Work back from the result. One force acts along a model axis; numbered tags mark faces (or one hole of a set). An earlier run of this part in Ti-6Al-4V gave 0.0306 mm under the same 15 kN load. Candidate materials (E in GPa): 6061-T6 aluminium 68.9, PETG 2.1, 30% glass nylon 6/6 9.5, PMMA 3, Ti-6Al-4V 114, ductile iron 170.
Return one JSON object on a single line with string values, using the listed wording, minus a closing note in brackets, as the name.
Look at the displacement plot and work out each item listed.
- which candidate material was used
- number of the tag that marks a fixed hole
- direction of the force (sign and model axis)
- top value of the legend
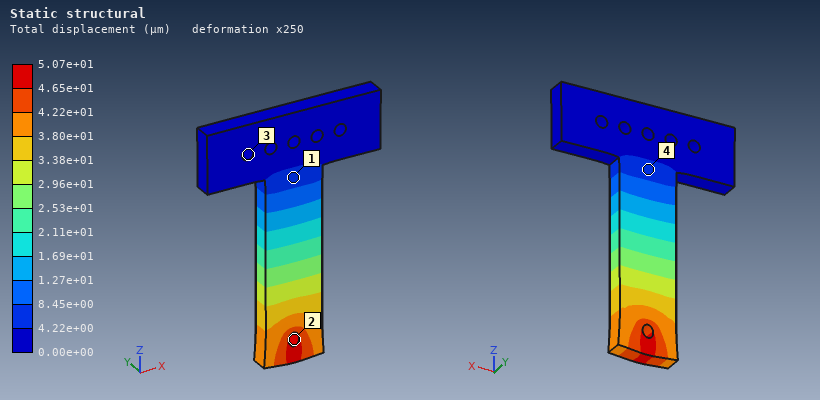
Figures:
{"which candidate material was used": "6061-T6 aluminium", "number of the tag that marks a fixed hole": "3", "direction of the force": "-Z", "top value of the legend": "5.07e+01 µm"}
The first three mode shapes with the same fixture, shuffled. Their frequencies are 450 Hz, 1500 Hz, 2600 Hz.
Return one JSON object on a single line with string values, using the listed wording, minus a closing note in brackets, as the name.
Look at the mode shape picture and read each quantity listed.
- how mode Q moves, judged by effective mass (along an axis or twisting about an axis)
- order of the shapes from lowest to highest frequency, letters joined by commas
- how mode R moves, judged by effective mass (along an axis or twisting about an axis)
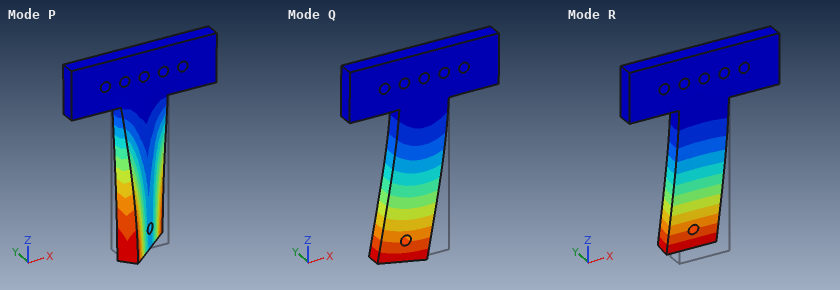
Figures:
{"how mode Q moves, judged by effective mass": "along X", "order of the shapes from lowest to highest frequency, letters joined by commas": "R, Q, P", "how mode R moves, judged by effective mass": "along Y"}
